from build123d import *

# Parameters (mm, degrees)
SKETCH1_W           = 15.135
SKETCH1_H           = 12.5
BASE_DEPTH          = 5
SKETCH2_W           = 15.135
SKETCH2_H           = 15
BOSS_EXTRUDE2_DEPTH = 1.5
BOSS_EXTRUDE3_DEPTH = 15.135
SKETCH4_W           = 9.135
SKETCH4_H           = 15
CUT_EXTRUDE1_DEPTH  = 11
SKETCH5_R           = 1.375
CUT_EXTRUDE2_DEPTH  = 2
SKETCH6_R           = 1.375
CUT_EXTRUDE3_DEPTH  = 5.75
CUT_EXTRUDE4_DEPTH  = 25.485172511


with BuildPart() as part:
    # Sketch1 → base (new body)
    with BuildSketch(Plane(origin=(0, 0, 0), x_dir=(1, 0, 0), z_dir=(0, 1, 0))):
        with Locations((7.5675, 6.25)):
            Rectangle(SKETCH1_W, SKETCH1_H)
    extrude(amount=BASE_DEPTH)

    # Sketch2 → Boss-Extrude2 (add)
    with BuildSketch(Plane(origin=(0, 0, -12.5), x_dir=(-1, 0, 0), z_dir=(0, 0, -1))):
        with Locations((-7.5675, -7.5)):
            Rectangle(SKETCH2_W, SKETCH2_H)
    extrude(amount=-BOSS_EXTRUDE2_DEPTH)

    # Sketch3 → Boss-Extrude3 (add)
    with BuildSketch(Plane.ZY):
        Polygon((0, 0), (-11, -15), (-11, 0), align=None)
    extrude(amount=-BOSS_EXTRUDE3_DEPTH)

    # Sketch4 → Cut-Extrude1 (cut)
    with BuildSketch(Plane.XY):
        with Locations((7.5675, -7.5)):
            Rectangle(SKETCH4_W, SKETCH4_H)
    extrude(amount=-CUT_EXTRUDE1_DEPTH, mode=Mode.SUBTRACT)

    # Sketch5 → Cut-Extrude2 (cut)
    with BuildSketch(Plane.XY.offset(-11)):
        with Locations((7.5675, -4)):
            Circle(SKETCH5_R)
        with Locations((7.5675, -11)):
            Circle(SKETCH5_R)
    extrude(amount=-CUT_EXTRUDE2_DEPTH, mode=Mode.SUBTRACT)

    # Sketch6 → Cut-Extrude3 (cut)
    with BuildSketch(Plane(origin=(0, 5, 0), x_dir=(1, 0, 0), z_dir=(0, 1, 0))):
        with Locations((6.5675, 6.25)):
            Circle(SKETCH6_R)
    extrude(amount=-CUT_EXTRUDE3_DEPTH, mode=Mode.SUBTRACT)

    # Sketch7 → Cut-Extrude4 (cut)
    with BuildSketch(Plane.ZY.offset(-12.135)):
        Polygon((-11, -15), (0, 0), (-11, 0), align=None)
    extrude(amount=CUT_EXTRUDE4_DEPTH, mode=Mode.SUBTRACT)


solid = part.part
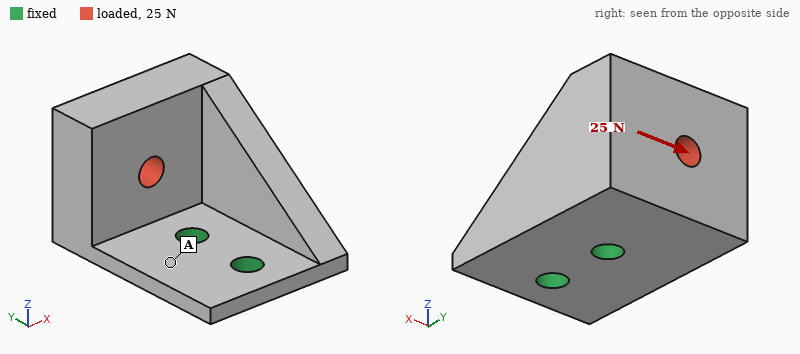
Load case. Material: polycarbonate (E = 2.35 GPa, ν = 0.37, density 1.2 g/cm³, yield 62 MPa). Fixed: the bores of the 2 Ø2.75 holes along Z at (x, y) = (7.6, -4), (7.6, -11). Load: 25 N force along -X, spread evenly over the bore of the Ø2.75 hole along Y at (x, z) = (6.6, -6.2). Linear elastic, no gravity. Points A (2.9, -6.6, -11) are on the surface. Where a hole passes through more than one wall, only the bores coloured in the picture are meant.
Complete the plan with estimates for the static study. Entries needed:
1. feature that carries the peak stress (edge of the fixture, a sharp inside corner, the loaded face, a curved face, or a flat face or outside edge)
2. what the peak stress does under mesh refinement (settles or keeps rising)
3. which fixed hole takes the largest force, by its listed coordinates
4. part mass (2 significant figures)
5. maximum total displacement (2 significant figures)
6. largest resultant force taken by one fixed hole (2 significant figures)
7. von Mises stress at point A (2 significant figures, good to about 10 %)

edge of the fixture
keeps rising
(7.6, -4)
1.8 g
0.28 mm
38 N
3.8 MPa
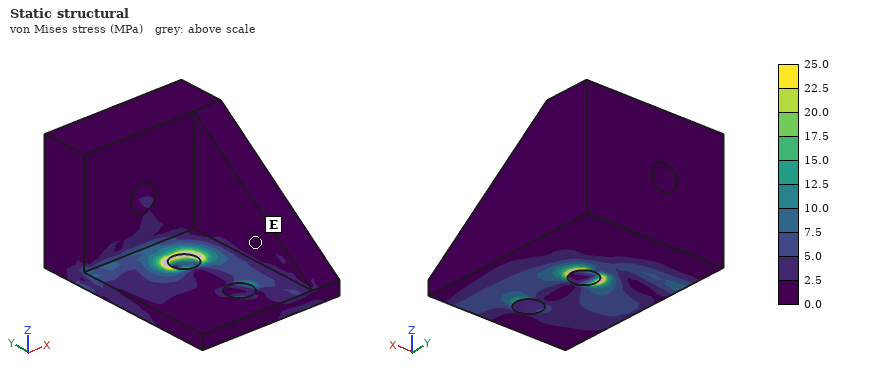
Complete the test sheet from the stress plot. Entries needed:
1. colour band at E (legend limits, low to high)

0.0 to 2.5 MPa
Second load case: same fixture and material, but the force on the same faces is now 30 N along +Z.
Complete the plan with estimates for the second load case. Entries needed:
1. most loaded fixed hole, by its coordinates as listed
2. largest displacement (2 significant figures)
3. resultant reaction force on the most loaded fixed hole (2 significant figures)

(7.6, -4)
0.19 mm
43 N
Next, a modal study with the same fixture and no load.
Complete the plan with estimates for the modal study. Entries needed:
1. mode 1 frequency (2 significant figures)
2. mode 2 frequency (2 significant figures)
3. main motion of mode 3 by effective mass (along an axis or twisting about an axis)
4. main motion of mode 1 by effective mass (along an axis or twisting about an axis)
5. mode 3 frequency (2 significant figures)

1400 Hz
2000 Hz
along Z
along X
5000 Hz
